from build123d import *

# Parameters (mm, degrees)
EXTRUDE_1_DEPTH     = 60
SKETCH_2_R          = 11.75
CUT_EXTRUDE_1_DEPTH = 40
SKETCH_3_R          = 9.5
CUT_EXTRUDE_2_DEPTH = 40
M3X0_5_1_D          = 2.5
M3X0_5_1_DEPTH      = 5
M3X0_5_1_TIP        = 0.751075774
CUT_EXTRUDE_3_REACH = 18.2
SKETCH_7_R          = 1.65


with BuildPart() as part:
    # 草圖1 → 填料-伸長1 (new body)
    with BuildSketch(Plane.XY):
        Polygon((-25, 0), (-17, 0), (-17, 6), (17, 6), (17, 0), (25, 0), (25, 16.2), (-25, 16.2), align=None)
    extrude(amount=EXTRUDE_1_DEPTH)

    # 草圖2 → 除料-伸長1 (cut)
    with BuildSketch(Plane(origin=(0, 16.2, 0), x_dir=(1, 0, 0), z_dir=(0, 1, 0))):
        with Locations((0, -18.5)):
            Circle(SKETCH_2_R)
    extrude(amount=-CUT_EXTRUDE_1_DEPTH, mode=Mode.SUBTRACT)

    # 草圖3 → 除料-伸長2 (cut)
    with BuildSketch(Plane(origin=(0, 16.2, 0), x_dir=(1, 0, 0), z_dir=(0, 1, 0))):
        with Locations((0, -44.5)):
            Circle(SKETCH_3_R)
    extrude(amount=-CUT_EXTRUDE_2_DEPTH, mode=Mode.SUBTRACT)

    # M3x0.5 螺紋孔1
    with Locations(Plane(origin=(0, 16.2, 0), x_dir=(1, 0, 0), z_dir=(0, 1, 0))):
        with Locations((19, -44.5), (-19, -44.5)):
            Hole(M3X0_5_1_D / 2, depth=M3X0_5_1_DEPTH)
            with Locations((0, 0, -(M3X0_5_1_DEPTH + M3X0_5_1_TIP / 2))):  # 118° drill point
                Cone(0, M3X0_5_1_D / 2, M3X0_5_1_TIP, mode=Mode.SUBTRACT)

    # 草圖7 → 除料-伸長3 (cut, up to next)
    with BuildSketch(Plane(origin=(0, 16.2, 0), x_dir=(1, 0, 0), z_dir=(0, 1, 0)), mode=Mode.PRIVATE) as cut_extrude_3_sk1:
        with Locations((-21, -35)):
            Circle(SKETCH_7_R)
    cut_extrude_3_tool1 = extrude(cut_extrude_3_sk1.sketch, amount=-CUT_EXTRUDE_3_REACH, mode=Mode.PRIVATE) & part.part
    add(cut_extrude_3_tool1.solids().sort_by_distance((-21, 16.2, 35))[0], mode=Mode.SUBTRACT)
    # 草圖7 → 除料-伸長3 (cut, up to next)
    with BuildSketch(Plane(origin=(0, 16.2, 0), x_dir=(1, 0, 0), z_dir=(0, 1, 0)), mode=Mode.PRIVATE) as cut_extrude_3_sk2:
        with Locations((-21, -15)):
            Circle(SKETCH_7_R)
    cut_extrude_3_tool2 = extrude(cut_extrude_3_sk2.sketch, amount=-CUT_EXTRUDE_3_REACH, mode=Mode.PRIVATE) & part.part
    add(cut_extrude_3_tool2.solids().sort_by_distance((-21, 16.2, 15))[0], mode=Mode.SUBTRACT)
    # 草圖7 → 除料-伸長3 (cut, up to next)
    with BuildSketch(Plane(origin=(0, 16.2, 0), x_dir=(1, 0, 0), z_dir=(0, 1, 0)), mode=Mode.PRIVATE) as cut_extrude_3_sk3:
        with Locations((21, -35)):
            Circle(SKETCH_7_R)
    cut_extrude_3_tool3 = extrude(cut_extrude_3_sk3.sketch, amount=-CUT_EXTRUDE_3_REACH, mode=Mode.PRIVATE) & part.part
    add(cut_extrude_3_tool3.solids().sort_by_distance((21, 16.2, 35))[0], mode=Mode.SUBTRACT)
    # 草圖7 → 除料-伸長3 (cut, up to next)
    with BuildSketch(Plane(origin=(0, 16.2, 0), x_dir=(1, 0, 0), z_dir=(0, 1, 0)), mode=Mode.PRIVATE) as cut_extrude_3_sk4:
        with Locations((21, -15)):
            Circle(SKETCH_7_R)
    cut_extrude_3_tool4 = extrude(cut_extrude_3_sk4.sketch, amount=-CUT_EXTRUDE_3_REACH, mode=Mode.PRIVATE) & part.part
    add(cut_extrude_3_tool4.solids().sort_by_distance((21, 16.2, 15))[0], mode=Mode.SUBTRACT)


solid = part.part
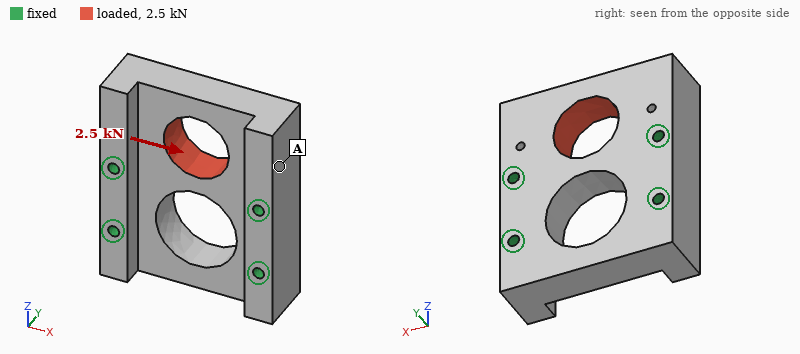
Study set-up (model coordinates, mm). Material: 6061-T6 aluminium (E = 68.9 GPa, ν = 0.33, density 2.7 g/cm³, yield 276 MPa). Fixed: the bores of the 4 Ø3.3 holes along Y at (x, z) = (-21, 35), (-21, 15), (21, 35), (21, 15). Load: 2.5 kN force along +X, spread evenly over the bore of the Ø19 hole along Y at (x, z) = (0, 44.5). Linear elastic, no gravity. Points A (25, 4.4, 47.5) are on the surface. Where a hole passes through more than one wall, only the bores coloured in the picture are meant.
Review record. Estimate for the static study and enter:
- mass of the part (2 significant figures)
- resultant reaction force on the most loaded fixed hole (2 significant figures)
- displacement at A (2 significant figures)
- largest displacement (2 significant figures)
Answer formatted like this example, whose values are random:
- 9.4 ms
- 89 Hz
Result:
- 77 g
- 1.4 kN
- 4.4 µm
- 8.2 µm
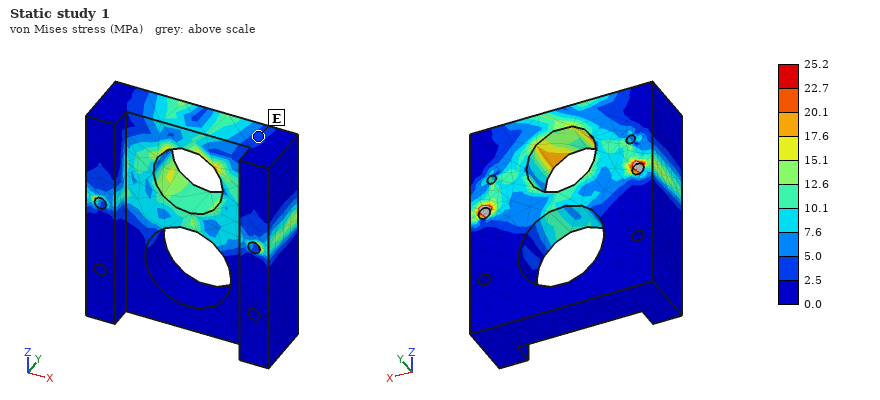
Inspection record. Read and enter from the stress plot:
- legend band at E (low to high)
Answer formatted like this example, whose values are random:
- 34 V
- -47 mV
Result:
- 2.5 to 5.0 MPa
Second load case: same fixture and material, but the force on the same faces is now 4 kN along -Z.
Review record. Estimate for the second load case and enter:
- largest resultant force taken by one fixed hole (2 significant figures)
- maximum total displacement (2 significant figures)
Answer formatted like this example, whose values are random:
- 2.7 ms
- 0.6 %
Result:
- 1.4 kN
- 8.5 µm
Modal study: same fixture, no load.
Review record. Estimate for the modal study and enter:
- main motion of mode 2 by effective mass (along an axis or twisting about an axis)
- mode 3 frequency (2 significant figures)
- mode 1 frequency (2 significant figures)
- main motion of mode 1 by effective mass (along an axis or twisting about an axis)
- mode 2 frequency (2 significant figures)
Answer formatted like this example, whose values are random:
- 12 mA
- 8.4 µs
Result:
- along X
- 18 kHz
- 12 kHz
- along Y
- 15 kHz
